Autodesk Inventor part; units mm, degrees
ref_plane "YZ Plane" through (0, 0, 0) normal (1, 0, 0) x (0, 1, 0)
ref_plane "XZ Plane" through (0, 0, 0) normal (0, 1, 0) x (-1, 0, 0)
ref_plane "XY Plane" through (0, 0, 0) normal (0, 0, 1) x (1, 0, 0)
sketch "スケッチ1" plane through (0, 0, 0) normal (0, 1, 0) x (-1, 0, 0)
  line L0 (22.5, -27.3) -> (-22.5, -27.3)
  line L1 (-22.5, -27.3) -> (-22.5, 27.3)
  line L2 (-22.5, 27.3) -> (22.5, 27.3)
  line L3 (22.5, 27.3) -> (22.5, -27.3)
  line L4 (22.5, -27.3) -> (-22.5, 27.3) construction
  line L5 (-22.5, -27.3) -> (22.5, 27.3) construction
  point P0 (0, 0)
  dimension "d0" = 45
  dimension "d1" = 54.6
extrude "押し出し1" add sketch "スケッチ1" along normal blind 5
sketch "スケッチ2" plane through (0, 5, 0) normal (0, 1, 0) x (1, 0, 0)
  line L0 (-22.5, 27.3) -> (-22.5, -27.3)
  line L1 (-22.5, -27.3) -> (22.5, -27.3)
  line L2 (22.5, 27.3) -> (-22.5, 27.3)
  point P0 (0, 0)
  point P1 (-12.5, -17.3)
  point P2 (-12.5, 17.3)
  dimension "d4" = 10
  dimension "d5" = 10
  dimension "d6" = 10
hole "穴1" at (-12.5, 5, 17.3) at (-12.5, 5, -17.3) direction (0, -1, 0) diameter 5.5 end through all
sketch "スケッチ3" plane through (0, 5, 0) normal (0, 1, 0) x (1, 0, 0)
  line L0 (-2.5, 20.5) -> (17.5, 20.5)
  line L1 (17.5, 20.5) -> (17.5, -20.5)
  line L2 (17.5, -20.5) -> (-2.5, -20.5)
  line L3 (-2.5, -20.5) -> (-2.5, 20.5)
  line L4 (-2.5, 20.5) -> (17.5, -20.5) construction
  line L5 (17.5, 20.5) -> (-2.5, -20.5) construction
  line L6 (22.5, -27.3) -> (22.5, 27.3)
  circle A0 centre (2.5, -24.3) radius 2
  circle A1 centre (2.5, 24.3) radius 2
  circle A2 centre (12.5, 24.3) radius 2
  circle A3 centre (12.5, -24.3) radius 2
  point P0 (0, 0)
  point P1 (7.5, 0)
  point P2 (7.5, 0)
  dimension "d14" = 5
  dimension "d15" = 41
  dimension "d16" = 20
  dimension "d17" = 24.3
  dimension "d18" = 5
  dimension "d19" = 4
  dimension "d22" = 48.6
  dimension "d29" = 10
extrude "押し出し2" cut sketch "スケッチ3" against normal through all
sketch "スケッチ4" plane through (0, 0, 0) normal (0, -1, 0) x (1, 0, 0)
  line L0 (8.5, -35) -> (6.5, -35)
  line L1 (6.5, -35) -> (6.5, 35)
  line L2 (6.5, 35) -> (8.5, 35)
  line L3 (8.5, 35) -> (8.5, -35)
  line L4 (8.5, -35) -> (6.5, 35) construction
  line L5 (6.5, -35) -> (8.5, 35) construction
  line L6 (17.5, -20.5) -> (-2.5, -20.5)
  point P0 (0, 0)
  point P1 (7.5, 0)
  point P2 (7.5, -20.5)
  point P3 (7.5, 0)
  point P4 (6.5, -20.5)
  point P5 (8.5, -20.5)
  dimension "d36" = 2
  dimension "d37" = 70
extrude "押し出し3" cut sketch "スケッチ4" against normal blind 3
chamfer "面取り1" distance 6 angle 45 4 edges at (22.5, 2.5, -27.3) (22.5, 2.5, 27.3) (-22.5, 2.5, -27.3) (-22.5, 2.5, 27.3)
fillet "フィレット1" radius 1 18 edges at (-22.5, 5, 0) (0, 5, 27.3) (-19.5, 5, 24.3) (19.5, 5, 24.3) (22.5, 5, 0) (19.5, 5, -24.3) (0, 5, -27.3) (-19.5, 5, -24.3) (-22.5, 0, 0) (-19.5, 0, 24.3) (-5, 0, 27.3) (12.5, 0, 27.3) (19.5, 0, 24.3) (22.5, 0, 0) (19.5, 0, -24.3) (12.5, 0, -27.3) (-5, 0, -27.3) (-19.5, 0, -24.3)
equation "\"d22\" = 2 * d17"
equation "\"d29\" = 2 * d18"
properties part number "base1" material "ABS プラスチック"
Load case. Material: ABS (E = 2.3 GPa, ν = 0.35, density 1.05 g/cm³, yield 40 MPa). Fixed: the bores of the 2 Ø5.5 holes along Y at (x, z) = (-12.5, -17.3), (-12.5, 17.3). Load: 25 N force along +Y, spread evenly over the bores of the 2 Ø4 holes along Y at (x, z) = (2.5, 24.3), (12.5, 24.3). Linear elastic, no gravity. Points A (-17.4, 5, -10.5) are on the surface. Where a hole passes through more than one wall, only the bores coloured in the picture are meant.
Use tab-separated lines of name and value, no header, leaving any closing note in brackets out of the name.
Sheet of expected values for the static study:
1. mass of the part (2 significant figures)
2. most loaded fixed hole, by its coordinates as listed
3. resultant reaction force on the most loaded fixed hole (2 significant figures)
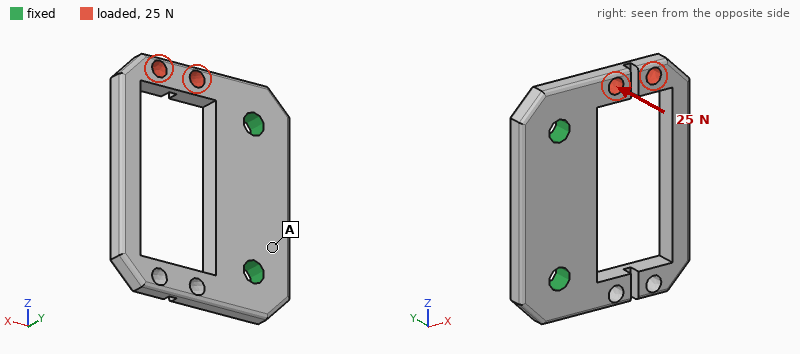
mass of the part	7.5 g
most loaded fixed hole, by its coordinates as listed	(-12.5, 17.3)
resultant reaction force on the most loaded fixed hole	26 N
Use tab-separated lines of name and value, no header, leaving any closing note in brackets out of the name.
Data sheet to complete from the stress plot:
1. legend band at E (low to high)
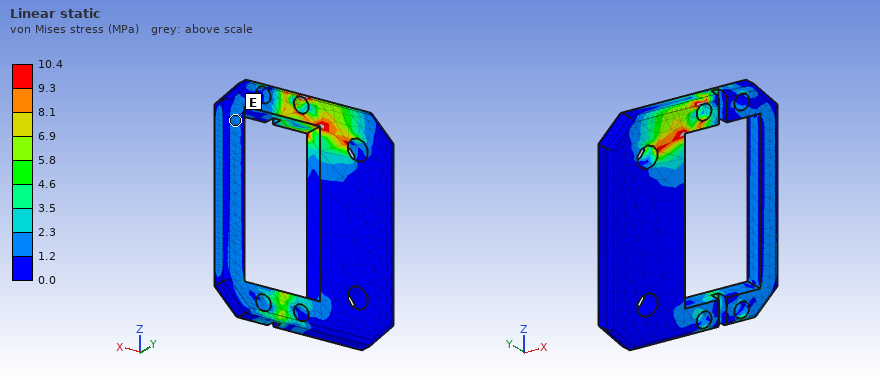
legend band at E	1.2 to 2.3 MPa
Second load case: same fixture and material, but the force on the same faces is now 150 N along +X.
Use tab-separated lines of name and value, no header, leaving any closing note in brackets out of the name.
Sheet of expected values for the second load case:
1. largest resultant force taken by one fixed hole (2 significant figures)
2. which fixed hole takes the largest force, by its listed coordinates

largest resultant force taken by one fixed hole	170 N
which fixed hole takes the largest force, by its listed coordinates	(-12.5, 17.3)
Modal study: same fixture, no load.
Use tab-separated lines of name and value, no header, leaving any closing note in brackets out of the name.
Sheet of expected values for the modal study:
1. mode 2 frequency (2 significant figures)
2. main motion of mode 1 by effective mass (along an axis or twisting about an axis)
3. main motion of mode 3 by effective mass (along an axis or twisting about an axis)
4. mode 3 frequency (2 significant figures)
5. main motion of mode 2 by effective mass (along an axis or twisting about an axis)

mode 2 frequency	1300 Hz
main motion of mode 1 by effective mass	along Y
main motion of mode 3 by effective mass	along Z
mode 3 frequency	1400 Hz
main motion of mode 2 by effective mass	twisting about X
